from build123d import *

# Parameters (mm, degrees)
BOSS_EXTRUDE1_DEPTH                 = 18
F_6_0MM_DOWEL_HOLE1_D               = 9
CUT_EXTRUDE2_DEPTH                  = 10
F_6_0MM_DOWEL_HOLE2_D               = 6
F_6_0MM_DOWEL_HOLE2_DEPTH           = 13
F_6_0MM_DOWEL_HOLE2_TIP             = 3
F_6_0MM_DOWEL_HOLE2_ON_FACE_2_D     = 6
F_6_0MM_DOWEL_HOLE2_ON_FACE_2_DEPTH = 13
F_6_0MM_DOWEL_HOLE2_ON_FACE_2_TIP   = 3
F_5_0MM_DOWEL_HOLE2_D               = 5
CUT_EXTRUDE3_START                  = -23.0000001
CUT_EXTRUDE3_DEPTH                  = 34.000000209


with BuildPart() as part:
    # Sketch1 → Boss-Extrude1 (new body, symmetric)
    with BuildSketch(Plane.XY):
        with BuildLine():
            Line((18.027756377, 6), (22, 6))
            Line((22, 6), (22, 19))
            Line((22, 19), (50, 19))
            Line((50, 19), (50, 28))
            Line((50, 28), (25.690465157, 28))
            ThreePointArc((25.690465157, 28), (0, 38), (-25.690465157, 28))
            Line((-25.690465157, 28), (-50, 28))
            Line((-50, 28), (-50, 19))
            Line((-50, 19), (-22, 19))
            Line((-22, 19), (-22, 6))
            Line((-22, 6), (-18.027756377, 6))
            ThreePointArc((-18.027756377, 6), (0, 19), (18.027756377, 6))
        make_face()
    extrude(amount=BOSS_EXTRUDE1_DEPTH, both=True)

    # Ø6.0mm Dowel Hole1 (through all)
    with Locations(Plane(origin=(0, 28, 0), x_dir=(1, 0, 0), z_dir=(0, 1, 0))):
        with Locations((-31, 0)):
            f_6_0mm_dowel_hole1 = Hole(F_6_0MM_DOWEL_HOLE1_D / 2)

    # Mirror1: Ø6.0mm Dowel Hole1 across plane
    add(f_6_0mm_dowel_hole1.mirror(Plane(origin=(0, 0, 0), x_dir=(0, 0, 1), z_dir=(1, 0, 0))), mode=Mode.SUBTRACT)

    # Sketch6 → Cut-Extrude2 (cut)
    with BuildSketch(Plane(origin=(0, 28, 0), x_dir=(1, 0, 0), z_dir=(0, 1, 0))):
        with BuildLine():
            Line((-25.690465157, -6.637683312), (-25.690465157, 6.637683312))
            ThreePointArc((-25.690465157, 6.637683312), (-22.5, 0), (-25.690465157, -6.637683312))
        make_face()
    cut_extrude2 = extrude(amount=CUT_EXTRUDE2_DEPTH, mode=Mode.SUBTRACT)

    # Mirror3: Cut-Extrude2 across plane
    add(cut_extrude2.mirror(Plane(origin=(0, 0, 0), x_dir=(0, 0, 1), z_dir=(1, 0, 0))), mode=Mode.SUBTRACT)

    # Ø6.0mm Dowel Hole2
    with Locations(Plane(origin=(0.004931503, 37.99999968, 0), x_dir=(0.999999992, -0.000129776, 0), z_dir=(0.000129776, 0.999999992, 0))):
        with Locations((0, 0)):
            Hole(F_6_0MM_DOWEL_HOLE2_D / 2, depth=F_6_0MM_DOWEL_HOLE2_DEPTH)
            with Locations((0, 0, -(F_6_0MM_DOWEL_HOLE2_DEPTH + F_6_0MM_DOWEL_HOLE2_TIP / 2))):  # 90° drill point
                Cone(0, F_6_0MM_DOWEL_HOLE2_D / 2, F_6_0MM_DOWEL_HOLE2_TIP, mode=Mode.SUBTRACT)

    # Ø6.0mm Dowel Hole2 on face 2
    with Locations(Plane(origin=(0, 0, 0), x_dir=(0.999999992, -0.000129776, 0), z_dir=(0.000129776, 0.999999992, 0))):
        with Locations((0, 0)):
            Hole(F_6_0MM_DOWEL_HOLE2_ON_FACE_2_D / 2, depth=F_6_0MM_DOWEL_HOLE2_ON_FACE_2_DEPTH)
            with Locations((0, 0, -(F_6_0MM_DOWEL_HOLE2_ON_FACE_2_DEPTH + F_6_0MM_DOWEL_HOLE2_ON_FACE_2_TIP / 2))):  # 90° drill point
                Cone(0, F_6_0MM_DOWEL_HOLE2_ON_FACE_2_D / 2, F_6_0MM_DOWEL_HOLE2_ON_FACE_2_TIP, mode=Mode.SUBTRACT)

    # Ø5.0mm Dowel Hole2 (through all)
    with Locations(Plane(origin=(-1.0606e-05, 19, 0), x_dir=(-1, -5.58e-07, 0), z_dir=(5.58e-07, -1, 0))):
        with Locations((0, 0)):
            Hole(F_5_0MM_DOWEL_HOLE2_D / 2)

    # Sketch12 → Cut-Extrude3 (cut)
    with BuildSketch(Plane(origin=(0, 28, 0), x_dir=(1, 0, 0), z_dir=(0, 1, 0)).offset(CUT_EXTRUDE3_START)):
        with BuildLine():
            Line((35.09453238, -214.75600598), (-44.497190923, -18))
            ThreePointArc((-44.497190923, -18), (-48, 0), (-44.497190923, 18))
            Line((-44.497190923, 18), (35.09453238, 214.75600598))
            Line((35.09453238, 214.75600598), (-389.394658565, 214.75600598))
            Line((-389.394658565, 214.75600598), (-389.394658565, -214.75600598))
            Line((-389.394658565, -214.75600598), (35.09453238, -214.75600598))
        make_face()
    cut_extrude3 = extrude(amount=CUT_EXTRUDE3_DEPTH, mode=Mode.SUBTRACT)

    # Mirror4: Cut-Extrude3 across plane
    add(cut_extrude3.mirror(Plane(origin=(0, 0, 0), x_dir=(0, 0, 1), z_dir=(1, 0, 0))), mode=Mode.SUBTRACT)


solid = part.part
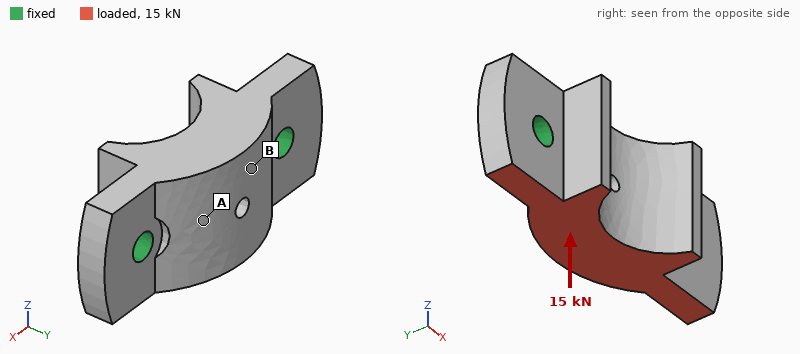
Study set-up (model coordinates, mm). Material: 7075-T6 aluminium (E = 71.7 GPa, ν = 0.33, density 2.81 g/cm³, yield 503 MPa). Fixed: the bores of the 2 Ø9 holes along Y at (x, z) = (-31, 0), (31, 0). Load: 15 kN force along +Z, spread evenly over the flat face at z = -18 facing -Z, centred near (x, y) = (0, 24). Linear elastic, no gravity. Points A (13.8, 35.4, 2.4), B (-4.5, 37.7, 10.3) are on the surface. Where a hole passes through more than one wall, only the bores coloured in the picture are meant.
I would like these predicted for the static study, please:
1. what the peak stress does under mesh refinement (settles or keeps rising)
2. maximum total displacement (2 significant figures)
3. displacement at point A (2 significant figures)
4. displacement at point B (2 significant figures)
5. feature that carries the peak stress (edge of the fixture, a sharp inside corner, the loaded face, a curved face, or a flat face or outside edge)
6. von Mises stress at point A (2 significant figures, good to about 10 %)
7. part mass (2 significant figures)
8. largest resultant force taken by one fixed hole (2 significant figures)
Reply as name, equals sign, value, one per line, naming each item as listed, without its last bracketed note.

what the peak stress does under mesh refinement = keeps rising
maximum total displacement = 22 µm
displacement at point A = 15 µm
displacement at point B = 18 µm
feature that carries the peak stress = edge of the fixture
von Mises stress at point A = 16 MPa
part mass = 140 g
largest resultant force taken by one fixed hole = 7.5 kN
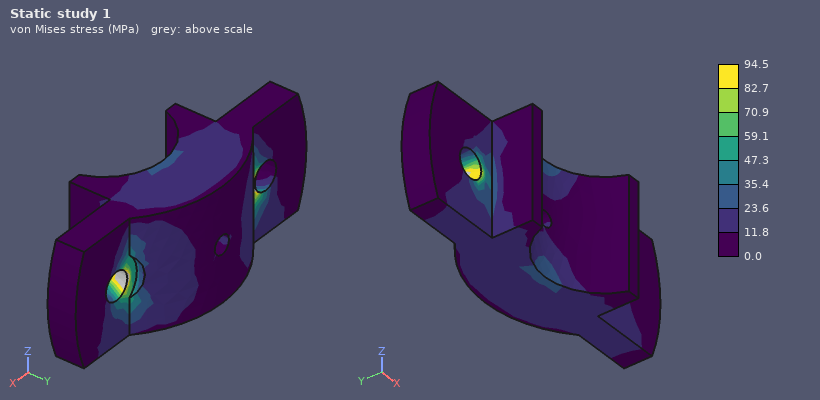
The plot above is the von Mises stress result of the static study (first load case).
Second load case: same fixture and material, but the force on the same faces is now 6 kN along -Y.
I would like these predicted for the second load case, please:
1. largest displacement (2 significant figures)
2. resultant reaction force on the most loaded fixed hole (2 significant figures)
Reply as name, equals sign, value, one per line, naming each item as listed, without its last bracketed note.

largest displacement = 52 µm
resultant reaction force on the most loaded fixed hole = 3.1 kN
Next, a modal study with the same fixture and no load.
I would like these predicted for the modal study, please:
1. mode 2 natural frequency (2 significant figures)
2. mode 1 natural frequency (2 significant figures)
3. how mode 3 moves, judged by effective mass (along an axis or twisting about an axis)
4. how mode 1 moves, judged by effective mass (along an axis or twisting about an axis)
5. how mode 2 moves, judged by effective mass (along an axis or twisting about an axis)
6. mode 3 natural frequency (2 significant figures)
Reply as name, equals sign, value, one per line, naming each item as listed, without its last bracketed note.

mode 2 natural frequency = 11 kHz
mode 1 natural frequency = 9000 Hz
how mode 3 moves, judged by effective mass = along Z
how mode 1 moves, judged by effective mass = twisting about X
how mode 2 moves, judged by effective mass = along Y
mode 3 natural frequency = 15 kHz
